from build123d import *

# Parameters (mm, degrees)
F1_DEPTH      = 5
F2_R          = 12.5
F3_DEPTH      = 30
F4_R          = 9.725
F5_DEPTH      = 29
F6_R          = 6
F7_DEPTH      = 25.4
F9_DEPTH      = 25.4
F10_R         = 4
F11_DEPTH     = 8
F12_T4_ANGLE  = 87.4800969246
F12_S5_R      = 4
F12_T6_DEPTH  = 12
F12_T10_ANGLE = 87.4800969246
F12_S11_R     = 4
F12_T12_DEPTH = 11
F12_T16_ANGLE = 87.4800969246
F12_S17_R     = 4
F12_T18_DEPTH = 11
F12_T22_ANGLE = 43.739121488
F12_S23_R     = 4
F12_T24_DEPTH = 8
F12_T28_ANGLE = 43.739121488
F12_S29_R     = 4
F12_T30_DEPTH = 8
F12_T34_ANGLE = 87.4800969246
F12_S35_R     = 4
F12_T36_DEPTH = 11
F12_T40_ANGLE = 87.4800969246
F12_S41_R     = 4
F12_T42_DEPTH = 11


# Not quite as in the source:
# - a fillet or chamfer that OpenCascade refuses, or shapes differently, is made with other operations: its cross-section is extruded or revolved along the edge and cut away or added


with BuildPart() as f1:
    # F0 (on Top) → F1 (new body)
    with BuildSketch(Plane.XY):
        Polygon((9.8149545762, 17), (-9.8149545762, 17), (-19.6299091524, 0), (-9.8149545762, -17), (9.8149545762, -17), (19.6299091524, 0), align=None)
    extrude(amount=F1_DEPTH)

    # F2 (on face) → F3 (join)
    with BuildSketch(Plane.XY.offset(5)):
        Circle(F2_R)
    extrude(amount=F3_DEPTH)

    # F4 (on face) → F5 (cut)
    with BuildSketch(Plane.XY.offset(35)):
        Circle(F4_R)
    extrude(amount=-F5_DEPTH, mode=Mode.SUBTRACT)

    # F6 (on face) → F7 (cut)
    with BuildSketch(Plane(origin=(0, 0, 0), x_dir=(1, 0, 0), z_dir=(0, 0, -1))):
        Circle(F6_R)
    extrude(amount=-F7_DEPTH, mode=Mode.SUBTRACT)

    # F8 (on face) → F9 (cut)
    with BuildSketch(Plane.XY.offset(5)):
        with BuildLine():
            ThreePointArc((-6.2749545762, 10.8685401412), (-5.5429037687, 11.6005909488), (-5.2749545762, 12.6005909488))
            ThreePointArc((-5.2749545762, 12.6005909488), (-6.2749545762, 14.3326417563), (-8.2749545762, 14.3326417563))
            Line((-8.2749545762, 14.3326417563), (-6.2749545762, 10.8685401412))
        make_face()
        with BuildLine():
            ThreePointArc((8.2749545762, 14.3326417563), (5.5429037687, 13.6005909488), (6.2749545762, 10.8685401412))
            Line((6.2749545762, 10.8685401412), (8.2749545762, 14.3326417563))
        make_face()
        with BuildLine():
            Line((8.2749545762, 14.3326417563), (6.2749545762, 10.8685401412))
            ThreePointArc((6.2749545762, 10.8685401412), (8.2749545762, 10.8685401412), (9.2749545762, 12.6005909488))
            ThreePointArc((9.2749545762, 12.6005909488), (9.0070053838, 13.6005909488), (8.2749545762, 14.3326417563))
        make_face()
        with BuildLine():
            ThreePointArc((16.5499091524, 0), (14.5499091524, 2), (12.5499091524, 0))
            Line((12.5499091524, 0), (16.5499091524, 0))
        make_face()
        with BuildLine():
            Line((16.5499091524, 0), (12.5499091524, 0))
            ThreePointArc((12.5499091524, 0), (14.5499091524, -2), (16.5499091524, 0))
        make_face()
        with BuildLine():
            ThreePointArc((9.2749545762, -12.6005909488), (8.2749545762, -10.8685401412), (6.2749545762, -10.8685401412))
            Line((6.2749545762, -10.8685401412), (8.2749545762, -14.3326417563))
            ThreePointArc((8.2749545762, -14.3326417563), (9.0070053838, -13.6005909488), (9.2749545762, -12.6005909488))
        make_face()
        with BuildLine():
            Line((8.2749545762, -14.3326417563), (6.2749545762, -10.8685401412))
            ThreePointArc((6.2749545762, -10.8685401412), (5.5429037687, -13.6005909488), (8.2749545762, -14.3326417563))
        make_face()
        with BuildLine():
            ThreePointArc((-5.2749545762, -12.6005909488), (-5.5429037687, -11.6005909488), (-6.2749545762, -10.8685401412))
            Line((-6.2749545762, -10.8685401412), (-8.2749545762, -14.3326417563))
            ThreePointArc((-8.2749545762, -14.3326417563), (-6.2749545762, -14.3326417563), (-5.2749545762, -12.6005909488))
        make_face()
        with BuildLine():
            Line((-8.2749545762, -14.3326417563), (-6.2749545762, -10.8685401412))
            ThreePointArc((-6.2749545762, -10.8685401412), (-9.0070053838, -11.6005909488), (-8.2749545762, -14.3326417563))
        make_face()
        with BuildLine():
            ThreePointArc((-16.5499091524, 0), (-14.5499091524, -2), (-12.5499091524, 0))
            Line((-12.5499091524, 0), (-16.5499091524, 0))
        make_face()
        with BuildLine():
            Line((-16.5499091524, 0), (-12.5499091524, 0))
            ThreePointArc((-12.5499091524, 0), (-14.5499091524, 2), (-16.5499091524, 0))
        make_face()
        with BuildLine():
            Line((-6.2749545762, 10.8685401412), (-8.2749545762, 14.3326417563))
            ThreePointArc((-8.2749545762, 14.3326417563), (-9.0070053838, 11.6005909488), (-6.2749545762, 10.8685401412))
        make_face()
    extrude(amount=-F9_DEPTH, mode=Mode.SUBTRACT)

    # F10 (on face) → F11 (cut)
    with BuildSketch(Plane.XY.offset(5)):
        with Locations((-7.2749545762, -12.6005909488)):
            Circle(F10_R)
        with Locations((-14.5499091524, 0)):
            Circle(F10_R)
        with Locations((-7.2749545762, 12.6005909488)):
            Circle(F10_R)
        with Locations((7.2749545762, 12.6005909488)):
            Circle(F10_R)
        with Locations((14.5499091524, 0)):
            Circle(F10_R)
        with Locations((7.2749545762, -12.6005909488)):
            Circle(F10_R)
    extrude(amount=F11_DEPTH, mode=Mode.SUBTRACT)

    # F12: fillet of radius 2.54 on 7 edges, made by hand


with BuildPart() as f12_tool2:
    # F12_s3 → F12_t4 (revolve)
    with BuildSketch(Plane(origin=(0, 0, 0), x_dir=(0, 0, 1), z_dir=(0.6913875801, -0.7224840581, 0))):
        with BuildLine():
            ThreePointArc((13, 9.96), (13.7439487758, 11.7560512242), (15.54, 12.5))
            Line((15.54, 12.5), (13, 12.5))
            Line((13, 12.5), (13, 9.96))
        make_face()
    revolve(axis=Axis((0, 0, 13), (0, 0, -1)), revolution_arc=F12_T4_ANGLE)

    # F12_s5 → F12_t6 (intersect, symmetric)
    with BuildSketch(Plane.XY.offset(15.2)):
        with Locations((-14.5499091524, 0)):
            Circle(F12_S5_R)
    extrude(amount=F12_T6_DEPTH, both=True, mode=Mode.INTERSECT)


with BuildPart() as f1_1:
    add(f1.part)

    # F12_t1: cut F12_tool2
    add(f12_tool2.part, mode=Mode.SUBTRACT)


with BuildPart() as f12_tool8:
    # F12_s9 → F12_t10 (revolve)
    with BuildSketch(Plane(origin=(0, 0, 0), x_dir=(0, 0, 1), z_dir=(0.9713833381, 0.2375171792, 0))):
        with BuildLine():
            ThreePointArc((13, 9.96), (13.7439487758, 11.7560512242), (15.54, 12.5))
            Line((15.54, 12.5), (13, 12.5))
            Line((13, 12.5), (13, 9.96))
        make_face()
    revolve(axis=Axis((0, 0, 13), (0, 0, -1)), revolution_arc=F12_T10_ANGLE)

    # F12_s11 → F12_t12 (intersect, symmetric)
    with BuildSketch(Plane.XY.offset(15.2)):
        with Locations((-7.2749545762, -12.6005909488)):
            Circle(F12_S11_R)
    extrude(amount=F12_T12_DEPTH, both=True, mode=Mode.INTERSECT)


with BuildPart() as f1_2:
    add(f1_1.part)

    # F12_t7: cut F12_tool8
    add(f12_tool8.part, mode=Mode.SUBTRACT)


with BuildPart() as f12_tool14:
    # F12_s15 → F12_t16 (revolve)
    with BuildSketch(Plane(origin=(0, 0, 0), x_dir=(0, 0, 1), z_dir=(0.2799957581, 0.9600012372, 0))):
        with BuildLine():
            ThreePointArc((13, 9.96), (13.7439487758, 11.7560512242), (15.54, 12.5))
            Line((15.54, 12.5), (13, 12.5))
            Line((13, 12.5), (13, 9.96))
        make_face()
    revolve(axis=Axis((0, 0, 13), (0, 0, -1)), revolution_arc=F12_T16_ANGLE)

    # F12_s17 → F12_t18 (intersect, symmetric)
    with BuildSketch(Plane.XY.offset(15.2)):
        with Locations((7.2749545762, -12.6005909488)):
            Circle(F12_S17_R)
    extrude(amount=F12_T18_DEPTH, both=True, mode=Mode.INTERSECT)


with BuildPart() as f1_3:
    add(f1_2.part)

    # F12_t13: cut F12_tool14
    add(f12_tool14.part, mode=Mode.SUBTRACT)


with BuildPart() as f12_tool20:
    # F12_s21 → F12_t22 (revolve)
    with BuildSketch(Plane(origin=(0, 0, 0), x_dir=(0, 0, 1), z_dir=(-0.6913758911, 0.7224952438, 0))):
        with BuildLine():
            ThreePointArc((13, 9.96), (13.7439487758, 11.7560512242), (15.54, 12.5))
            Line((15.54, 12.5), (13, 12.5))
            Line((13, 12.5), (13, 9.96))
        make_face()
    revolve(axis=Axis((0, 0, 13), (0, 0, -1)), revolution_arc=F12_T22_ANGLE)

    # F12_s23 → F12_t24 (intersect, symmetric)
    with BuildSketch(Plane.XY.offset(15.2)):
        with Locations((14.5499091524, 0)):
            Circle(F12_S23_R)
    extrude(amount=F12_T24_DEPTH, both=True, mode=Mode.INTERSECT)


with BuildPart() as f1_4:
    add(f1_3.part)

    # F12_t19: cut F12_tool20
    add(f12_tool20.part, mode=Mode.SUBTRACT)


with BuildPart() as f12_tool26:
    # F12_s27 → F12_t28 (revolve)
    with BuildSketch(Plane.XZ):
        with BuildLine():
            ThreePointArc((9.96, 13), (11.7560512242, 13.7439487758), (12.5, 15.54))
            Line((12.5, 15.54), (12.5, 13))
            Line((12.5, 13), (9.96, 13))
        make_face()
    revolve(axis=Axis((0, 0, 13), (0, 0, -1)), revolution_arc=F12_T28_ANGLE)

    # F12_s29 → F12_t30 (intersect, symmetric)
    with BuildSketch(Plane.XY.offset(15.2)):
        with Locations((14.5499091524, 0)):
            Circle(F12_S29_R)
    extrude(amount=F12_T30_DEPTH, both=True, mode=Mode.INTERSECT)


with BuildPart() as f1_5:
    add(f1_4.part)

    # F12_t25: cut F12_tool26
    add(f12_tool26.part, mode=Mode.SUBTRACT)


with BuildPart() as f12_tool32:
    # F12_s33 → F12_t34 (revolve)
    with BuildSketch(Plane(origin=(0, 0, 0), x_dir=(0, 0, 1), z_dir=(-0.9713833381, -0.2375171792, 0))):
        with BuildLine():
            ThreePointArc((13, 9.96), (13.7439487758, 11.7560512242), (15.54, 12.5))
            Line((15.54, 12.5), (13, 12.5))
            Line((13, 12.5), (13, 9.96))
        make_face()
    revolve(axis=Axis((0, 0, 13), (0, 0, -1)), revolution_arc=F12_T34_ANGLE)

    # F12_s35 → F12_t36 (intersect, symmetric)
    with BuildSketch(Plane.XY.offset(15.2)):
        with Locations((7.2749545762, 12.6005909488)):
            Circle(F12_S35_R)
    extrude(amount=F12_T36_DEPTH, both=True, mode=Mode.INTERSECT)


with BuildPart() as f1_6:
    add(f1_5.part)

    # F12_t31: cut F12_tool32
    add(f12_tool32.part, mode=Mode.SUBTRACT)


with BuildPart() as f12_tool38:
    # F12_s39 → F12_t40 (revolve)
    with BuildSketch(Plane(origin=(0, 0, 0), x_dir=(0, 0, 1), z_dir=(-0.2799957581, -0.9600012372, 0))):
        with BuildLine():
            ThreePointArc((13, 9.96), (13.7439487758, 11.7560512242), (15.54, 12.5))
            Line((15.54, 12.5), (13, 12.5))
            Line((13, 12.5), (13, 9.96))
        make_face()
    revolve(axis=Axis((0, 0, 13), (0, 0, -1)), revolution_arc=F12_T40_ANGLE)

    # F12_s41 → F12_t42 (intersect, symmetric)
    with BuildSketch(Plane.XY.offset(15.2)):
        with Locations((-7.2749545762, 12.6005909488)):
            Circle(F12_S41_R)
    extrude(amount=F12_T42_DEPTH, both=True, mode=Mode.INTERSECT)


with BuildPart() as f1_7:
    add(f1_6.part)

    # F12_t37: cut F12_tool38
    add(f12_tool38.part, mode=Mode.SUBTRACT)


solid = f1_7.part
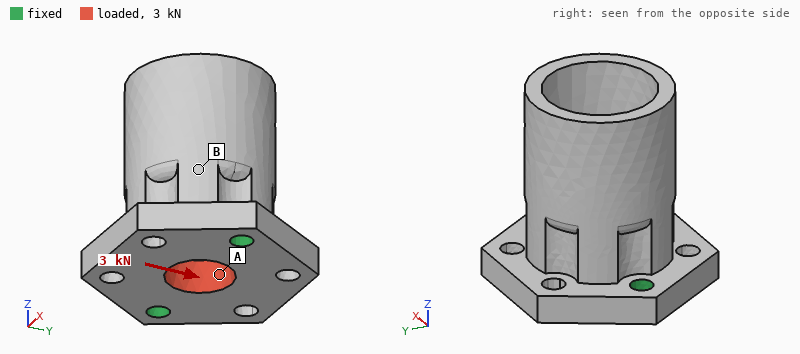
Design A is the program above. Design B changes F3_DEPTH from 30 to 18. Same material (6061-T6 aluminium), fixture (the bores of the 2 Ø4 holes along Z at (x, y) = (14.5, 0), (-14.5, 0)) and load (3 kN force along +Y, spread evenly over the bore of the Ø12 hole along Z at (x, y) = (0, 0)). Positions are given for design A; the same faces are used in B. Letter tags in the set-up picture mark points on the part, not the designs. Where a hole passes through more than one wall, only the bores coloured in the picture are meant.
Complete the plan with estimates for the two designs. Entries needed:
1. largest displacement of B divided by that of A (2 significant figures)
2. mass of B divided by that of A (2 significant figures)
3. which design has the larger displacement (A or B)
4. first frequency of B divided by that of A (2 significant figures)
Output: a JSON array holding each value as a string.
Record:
["0.76", "0.76", "A", "1.7"]
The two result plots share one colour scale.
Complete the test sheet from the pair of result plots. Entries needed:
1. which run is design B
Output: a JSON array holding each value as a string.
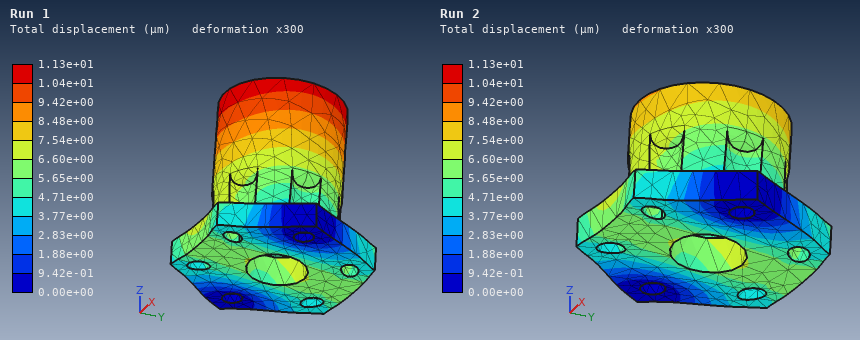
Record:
["Run 2"]
